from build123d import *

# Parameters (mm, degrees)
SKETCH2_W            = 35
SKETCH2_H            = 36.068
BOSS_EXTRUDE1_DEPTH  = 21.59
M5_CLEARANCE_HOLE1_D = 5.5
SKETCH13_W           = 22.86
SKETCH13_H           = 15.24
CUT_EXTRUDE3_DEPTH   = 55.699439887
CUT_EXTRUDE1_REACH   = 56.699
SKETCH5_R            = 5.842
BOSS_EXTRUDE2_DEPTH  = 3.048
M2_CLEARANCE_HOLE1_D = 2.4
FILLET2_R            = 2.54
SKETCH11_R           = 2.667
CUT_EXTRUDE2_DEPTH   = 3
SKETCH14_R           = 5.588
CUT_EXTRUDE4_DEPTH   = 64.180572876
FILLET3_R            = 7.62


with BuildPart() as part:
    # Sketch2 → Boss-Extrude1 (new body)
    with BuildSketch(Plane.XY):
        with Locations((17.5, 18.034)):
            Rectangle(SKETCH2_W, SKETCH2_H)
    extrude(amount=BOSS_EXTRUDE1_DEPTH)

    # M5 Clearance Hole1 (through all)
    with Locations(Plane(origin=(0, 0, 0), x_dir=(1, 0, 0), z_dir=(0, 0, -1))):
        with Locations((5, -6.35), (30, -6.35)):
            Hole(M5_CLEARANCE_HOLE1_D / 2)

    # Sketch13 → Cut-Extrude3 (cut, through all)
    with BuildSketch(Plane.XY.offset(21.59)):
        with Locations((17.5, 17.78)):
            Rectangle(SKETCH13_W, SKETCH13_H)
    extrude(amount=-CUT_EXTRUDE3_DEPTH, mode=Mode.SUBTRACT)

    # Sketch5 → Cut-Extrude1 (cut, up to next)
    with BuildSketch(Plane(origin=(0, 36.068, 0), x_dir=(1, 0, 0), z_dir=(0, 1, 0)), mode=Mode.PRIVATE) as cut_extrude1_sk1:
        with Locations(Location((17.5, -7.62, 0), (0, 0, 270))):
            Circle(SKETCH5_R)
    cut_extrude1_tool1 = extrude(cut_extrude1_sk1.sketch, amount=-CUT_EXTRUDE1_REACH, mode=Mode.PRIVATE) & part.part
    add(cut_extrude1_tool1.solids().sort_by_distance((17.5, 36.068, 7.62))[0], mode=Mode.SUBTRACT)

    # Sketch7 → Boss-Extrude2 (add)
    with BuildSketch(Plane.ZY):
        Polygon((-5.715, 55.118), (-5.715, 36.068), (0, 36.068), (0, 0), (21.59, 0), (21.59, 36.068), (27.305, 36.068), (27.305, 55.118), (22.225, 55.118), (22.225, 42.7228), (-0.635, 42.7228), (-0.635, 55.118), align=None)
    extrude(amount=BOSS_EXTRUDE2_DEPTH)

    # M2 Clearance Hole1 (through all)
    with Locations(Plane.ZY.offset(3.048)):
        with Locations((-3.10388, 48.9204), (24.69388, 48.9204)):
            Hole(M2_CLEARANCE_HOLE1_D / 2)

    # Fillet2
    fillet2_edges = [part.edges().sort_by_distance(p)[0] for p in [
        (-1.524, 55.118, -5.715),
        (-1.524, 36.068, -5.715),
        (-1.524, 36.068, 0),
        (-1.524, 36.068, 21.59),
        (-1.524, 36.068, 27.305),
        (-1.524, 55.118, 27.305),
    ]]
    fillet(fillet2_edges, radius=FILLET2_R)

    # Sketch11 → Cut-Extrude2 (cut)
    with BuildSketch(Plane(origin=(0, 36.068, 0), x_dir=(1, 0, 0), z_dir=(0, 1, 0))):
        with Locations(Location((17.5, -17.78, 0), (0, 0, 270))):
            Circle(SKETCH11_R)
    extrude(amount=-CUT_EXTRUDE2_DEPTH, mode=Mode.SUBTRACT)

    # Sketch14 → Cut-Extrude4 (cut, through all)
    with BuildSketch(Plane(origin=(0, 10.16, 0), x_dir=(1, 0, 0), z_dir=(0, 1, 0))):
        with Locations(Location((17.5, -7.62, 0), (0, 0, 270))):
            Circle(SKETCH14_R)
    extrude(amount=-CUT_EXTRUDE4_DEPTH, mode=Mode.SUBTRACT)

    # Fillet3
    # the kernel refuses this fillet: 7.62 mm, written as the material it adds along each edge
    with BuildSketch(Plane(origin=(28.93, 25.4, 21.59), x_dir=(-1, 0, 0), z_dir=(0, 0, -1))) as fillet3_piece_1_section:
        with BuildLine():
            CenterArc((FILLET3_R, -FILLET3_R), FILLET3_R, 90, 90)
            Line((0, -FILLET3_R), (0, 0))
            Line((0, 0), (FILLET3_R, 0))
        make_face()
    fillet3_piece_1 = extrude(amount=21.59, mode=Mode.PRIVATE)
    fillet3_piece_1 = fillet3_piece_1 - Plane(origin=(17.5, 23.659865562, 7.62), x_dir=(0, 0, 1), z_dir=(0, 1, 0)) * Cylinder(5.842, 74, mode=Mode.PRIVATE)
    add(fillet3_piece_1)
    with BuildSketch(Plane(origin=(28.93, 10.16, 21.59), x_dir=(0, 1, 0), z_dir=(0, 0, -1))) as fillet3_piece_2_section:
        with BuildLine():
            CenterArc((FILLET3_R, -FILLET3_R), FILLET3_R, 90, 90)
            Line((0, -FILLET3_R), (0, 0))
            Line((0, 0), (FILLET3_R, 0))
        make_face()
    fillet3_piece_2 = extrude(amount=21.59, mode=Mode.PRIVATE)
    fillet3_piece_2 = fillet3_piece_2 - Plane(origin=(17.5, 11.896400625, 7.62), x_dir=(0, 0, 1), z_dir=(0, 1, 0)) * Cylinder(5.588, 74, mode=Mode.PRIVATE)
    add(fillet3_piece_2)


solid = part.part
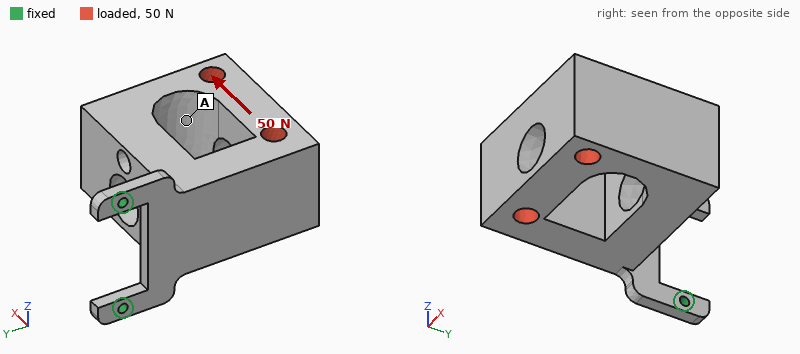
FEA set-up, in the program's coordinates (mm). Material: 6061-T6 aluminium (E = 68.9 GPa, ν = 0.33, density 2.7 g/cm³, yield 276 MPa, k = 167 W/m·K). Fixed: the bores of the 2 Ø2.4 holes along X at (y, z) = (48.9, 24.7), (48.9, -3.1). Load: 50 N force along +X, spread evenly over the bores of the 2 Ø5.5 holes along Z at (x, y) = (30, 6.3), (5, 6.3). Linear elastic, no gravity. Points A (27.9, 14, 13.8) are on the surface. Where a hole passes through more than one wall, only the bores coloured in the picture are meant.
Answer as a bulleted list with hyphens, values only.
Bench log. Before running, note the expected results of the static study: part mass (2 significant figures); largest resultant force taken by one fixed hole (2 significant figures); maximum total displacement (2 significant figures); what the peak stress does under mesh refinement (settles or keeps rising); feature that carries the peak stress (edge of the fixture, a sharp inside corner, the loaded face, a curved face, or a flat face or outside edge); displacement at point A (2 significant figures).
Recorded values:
- 55 g
- 25 N
- 0.73 mm
- keeps rising
- edge of the fixture
- 0.53 mm
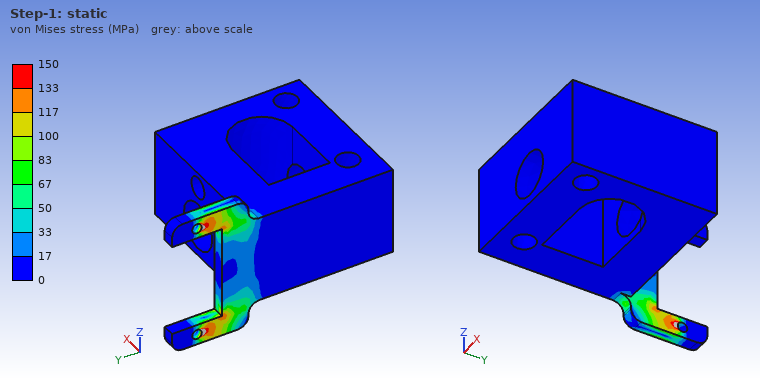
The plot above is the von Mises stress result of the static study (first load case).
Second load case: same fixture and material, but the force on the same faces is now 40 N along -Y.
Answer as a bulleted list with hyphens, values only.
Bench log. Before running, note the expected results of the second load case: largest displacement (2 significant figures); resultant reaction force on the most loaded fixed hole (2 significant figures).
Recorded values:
- 0.31 mm
- 21 N
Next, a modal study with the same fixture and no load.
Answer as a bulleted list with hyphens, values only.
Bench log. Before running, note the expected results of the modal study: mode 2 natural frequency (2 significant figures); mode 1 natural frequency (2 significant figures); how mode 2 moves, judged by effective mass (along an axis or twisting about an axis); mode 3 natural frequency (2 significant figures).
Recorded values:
- 1000 Hz
- 240 Hz
- along Z
- 2400 Hz
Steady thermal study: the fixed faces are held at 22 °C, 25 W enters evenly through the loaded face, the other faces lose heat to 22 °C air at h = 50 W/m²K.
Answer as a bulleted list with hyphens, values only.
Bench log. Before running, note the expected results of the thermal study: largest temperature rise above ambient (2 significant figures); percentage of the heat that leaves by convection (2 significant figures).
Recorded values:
- 42 K
- 53 %
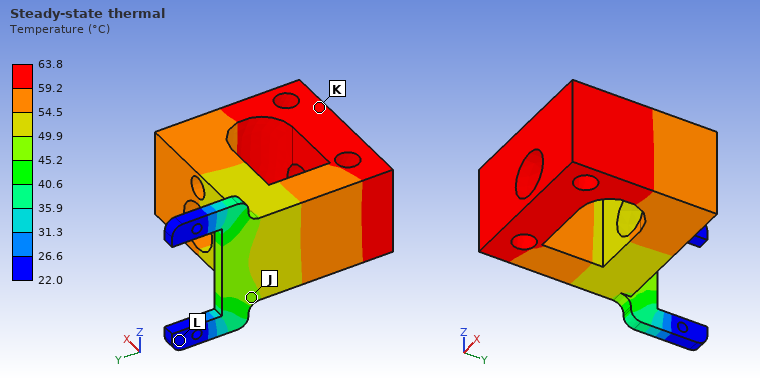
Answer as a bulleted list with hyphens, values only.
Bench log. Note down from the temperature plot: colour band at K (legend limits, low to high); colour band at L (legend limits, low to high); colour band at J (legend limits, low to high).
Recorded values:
- 59.2 to 63.8 °C
- 22.0 to 26.6 °C
- 45.2 to 49.9 °C
